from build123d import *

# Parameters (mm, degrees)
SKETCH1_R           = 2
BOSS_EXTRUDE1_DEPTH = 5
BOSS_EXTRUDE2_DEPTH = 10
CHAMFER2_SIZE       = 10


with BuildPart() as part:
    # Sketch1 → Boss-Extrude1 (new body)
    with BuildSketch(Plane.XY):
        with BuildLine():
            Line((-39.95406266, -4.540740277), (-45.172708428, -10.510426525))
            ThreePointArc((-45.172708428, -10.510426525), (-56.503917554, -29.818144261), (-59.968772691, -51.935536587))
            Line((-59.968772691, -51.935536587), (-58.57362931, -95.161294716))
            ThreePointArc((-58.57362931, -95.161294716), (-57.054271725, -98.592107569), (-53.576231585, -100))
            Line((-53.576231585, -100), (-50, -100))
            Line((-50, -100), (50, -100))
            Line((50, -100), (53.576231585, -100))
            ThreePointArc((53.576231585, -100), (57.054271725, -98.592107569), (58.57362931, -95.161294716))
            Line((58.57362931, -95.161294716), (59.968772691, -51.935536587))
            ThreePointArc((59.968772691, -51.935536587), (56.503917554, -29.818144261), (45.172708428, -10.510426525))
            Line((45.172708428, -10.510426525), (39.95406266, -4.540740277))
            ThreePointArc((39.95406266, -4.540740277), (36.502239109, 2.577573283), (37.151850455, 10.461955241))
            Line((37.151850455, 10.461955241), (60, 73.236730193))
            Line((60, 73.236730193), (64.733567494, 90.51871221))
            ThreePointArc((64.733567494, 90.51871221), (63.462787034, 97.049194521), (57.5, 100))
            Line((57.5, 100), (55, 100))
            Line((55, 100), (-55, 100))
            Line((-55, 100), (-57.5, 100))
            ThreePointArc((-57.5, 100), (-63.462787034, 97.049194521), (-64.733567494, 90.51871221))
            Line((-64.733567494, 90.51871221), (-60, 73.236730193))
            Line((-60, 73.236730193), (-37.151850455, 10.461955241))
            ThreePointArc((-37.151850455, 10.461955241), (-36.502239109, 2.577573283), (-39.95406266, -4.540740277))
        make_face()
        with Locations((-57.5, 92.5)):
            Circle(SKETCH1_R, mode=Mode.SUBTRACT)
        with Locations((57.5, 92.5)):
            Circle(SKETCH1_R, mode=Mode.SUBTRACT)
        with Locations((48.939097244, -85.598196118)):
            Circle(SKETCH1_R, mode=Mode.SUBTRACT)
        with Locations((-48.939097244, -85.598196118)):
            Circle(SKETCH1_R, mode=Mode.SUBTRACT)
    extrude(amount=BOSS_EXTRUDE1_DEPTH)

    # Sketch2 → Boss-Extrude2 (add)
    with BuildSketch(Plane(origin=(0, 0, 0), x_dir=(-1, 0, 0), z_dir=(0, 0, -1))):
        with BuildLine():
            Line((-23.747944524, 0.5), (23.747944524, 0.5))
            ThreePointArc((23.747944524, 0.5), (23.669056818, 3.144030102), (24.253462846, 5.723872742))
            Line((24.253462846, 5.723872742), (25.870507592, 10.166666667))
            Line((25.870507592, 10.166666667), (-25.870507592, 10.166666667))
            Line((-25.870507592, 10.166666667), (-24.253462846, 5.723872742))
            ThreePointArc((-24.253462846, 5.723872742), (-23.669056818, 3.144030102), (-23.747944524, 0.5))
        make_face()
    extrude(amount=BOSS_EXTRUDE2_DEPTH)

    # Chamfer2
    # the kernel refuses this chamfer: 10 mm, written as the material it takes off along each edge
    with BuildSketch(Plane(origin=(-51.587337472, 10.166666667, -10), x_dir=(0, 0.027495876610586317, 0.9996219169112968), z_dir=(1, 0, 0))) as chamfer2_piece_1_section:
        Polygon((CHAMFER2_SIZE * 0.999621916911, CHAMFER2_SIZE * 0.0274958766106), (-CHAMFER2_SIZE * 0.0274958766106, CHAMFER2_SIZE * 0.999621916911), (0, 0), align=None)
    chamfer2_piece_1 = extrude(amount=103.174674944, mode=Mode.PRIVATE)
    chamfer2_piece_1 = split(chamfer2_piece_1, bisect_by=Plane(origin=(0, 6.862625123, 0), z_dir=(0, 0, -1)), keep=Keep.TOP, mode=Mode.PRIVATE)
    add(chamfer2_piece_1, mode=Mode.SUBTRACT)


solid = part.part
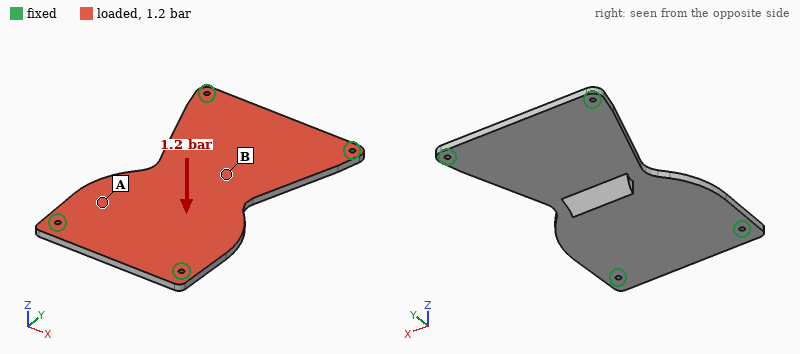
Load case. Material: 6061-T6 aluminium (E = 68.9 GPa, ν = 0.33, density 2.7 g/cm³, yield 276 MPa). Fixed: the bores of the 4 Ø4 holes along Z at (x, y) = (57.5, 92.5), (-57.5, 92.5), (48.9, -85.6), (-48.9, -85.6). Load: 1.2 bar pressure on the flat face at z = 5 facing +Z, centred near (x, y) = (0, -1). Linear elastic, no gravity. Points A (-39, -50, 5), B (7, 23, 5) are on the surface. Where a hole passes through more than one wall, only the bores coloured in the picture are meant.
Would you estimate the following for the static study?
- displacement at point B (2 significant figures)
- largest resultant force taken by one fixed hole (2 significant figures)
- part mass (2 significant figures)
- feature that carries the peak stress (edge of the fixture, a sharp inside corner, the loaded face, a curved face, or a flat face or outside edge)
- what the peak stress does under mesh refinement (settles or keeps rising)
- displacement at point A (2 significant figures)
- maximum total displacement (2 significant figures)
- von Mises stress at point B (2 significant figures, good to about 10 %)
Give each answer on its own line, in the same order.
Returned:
0.67 mm
690 N
290 g
edge of the fixture
keeps rising
0.32 mm
0.71 mm
42 MPa
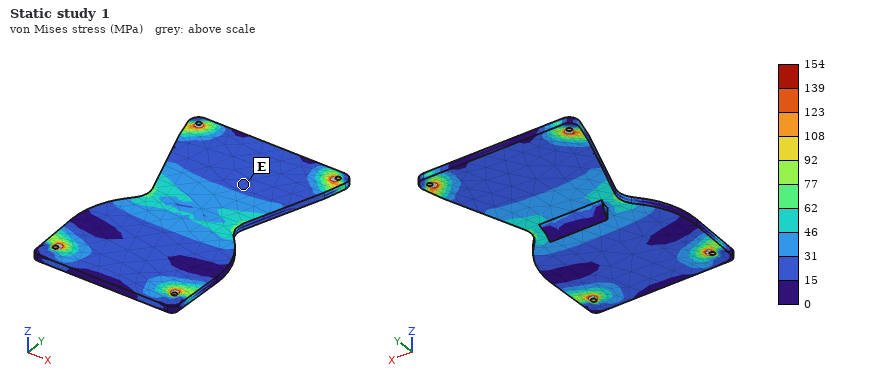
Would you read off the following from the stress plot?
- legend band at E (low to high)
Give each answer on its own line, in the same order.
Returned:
15 to 31 MPa
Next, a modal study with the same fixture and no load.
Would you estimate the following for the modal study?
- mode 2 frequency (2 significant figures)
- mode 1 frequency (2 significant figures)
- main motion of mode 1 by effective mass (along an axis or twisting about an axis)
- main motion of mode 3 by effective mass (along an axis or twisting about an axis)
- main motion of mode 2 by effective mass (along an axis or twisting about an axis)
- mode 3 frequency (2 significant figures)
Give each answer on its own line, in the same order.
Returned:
1400 Hz
640 Hz
along Z
twisting about X
twisting about Y
1600 Hz
